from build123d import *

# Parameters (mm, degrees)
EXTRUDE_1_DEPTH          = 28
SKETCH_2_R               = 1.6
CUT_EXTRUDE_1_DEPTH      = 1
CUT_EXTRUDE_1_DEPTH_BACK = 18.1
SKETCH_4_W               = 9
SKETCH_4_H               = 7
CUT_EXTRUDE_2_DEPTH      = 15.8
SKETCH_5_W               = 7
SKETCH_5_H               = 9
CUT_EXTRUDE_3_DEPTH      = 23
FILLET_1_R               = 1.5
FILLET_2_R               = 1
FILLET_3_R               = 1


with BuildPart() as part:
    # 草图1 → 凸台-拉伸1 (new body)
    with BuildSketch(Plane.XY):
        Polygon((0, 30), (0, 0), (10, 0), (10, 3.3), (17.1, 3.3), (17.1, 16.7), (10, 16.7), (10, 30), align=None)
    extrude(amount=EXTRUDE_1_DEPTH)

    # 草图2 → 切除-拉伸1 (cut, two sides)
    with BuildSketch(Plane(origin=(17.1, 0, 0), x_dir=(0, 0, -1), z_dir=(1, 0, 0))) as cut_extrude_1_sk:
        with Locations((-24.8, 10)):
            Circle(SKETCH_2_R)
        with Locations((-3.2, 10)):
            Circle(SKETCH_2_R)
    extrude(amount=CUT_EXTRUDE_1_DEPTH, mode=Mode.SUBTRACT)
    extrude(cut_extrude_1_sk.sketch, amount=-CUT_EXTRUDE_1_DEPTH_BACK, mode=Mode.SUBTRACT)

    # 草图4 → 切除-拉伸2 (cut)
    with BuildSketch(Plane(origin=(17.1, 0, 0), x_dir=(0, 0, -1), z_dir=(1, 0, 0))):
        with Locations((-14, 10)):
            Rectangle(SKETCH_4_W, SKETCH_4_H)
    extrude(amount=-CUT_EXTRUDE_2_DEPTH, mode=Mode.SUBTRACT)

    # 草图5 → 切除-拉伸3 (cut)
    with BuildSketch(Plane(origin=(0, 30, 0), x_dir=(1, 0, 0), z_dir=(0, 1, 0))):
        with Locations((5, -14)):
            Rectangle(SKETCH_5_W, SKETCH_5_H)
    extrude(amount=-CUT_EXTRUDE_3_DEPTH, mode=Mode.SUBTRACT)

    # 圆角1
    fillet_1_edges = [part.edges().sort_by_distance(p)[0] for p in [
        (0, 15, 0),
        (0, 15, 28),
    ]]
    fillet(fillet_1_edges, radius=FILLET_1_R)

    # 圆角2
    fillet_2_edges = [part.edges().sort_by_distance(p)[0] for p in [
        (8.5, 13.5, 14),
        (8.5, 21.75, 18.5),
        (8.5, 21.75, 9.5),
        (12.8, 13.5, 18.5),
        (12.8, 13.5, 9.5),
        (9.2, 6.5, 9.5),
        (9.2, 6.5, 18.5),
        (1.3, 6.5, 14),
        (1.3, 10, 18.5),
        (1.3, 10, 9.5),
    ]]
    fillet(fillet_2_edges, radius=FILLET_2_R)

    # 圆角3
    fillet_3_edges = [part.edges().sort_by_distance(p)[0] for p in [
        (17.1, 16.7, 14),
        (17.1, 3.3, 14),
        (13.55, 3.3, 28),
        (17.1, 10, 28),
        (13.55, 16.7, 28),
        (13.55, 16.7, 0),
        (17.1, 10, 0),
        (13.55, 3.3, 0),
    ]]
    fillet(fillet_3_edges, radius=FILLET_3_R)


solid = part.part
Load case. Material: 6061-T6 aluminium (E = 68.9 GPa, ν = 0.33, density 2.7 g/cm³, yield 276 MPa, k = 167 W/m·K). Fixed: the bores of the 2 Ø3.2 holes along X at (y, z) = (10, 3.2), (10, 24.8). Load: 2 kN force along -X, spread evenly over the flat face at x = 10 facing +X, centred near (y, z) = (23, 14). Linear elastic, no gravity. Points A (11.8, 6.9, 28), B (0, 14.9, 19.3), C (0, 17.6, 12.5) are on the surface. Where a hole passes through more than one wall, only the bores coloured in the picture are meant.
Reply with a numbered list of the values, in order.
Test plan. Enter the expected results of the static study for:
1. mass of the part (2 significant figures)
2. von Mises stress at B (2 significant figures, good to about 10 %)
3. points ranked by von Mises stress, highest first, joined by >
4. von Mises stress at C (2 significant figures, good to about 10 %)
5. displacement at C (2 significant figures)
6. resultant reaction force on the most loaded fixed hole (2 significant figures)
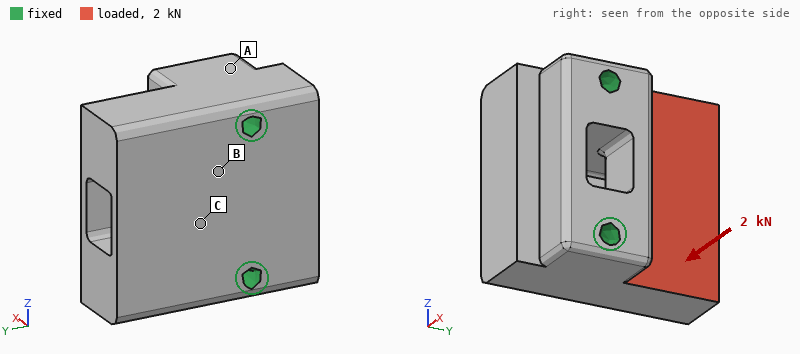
1. 24 g
2. 24 MPa
3. B > C > A
4. 14 MPa
5. 6.5 µm
6. 1.0 kN
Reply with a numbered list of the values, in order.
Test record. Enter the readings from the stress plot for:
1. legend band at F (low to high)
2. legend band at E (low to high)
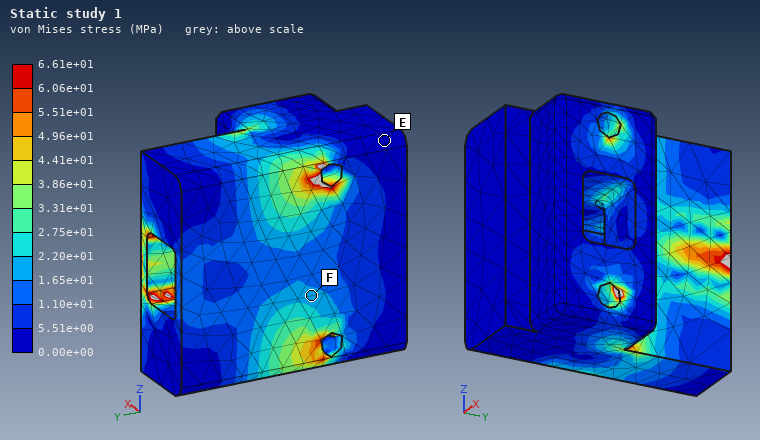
1. 1.65e+01 to 2.20e+01 MPa
2. 0.00e+00 to 5.51e+00 MPa
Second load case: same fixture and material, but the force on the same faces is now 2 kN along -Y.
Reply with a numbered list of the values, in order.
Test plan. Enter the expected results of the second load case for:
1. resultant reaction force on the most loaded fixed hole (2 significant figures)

1. 1.0 kN
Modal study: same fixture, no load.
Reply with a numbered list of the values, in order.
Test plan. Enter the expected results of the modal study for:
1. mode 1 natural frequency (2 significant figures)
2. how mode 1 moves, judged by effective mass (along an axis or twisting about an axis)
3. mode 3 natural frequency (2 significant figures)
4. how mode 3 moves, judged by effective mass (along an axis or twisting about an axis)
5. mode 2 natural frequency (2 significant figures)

1. 21 kHz
2. along X
3. 28 kHz
4. along Z
5. 26 kHz
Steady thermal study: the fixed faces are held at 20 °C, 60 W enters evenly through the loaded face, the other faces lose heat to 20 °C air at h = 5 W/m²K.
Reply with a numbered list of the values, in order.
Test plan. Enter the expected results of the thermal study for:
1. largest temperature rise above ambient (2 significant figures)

1. 31 K
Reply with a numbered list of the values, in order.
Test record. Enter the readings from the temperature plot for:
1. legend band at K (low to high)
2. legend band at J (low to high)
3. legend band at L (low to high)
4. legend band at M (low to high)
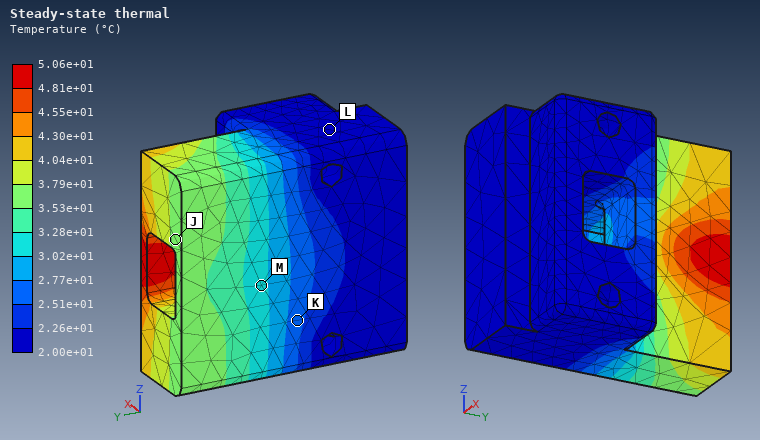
1. 2.51e+01 to 2.77e+01 °C
2. 3.53e+01 to 3.79e+01 °C
3. 2.00e+01 to 2.26e+01 °C
4. 3.02e+01 to 3.28e+01 °C
